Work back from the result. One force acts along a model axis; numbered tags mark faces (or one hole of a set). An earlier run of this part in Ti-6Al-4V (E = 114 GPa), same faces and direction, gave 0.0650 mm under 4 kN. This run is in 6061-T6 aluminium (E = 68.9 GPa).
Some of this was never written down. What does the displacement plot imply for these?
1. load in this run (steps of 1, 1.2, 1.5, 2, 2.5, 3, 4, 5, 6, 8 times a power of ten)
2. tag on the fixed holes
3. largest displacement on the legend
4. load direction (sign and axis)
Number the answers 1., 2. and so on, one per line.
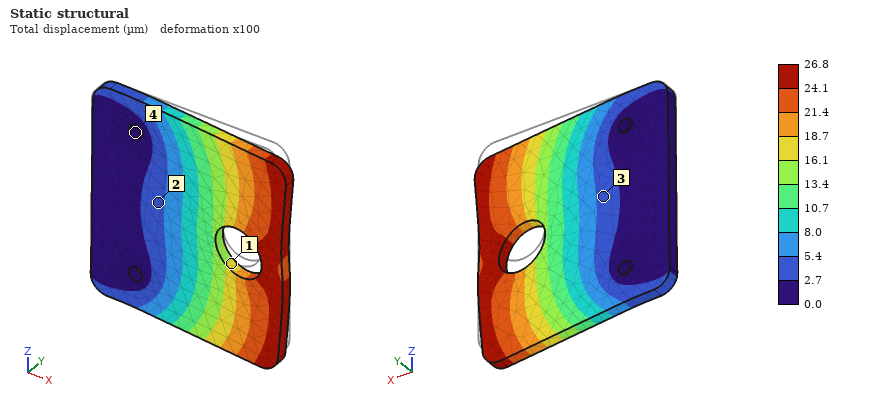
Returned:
1. 1 kN
2. 4
3. 26.8 µm
4. -Z
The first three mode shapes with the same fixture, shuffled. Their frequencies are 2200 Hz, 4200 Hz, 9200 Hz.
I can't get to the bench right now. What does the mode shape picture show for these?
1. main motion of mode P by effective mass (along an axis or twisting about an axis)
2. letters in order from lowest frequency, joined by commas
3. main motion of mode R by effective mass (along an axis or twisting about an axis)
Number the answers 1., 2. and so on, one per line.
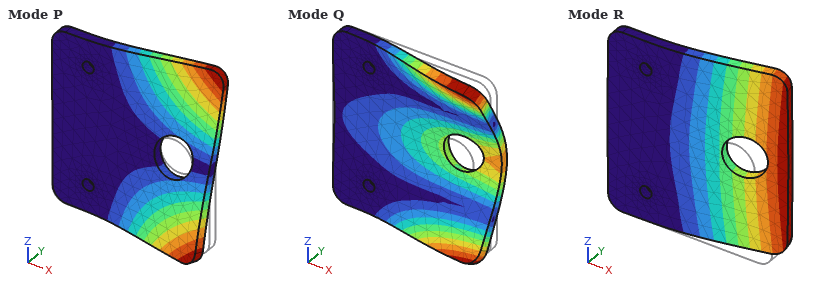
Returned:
1. twisting about X
2. R, P, Q
3. along Y
